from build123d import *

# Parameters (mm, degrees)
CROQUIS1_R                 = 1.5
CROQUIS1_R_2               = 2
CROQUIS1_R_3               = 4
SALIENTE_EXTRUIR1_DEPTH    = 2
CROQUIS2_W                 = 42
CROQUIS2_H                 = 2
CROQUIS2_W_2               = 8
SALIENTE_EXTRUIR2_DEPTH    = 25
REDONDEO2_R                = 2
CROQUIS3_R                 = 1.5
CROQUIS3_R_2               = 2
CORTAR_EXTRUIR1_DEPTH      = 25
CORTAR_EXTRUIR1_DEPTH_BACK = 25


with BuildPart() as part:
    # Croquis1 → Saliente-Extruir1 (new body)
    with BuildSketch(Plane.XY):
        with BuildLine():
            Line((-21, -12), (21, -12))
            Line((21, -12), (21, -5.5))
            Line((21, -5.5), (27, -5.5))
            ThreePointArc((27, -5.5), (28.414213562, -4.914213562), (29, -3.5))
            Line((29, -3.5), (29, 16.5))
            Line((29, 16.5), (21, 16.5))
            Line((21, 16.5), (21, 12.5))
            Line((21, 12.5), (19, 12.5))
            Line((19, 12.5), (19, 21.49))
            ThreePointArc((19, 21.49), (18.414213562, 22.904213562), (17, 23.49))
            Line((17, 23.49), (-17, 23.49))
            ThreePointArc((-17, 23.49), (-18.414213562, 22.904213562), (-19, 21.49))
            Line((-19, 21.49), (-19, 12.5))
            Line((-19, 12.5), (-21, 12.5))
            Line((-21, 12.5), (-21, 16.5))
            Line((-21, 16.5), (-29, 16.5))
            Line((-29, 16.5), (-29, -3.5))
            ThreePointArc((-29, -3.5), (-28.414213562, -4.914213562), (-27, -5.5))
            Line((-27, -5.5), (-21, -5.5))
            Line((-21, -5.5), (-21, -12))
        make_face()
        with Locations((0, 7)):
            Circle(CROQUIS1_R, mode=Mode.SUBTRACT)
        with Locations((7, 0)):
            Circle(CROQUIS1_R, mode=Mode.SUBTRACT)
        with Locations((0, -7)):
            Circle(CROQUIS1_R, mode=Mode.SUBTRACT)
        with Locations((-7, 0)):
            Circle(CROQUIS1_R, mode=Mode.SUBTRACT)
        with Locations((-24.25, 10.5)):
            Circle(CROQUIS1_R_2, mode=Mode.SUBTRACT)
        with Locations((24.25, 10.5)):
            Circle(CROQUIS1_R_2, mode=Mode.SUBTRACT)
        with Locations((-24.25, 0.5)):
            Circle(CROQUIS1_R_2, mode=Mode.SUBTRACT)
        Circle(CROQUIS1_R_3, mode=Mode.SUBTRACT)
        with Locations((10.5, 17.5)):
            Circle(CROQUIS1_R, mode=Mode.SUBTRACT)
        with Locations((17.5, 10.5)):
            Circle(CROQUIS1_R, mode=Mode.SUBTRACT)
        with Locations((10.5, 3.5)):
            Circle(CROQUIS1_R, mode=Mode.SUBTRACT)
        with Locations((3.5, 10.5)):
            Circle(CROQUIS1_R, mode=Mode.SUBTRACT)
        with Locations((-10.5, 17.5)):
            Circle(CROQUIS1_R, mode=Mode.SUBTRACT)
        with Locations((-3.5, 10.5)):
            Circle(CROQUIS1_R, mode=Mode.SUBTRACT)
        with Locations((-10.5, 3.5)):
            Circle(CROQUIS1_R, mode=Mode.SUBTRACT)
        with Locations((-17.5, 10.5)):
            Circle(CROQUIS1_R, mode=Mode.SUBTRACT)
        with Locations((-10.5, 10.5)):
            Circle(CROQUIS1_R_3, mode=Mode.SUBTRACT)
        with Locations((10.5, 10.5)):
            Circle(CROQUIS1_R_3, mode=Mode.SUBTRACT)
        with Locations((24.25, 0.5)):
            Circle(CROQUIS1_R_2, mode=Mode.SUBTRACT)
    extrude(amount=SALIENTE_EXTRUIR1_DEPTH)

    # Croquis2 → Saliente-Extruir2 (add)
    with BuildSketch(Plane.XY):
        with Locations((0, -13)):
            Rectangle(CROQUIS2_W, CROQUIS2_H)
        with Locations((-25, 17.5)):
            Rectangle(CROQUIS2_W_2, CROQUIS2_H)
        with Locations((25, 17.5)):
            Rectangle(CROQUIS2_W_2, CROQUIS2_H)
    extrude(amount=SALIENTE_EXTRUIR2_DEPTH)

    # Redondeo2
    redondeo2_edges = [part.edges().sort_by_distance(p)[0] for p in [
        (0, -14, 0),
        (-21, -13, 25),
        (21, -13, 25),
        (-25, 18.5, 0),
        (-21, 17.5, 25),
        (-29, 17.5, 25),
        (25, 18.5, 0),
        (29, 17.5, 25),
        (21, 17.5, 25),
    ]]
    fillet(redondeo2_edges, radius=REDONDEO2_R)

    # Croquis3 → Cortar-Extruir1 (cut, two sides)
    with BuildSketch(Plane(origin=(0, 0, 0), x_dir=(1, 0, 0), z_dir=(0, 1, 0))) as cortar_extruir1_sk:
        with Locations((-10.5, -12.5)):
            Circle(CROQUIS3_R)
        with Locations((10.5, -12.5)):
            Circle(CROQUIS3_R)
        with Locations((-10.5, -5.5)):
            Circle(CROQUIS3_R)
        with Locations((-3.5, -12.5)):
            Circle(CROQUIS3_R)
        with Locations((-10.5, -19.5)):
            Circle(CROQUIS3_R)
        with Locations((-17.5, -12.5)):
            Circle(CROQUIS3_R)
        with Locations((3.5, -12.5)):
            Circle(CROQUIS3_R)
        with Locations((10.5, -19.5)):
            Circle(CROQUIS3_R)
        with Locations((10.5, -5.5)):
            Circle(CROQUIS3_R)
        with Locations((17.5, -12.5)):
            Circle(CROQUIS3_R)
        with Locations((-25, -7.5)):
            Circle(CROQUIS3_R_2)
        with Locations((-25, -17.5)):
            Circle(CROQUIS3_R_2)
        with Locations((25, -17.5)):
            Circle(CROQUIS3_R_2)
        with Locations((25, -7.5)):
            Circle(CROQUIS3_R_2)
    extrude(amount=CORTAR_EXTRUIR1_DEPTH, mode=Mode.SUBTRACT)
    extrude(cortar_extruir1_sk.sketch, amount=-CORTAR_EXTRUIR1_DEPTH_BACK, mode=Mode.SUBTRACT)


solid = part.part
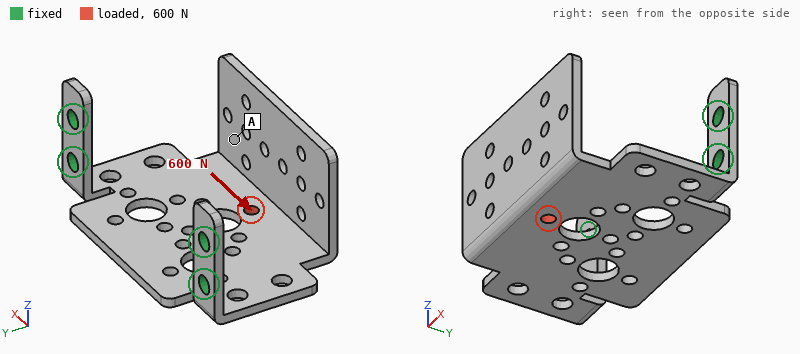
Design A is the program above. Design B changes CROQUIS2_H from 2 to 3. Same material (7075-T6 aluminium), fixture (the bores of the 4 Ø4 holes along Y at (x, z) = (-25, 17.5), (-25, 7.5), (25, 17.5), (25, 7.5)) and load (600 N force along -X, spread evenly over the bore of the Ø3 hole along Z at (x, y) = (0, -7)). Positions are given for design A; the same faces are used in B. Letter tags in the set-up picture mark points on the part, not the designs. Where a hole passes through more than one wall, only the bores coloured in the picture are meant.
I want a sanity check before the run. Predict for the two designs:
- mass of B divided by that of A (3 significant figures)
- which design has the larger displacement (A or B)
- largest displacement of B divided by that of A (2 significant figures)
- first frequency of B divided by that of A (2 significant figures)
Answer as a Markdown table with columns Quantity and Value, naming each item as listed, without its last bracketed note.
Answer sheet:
| Quantity | Value |
|---|---|
| mass of B divided by that of A | 1.23 |
| which design has the larger displacement | A |
| largest displacement of B divided by that of A | 0.48 |
| first frequency of B divided by that of A | 0.97 |
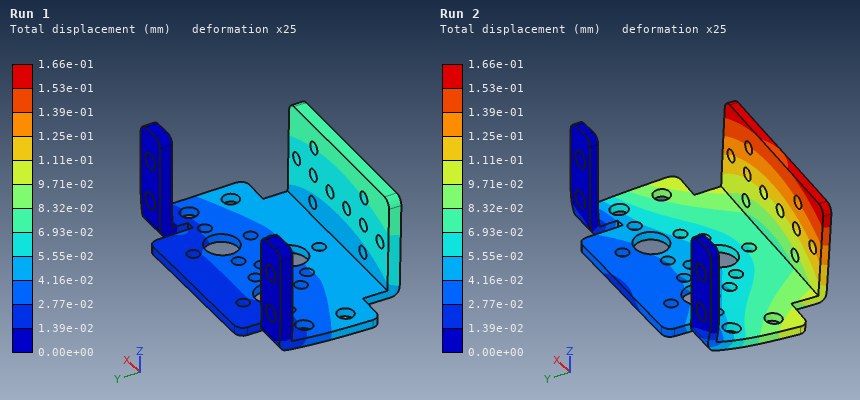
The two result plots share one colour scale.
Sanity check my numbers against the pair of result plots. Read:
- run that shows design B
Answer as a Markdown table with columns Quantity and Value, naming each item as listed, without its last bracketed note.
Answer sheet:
| Quantity | Value |
|---|---|
| run that shows design B | Run 1 |
